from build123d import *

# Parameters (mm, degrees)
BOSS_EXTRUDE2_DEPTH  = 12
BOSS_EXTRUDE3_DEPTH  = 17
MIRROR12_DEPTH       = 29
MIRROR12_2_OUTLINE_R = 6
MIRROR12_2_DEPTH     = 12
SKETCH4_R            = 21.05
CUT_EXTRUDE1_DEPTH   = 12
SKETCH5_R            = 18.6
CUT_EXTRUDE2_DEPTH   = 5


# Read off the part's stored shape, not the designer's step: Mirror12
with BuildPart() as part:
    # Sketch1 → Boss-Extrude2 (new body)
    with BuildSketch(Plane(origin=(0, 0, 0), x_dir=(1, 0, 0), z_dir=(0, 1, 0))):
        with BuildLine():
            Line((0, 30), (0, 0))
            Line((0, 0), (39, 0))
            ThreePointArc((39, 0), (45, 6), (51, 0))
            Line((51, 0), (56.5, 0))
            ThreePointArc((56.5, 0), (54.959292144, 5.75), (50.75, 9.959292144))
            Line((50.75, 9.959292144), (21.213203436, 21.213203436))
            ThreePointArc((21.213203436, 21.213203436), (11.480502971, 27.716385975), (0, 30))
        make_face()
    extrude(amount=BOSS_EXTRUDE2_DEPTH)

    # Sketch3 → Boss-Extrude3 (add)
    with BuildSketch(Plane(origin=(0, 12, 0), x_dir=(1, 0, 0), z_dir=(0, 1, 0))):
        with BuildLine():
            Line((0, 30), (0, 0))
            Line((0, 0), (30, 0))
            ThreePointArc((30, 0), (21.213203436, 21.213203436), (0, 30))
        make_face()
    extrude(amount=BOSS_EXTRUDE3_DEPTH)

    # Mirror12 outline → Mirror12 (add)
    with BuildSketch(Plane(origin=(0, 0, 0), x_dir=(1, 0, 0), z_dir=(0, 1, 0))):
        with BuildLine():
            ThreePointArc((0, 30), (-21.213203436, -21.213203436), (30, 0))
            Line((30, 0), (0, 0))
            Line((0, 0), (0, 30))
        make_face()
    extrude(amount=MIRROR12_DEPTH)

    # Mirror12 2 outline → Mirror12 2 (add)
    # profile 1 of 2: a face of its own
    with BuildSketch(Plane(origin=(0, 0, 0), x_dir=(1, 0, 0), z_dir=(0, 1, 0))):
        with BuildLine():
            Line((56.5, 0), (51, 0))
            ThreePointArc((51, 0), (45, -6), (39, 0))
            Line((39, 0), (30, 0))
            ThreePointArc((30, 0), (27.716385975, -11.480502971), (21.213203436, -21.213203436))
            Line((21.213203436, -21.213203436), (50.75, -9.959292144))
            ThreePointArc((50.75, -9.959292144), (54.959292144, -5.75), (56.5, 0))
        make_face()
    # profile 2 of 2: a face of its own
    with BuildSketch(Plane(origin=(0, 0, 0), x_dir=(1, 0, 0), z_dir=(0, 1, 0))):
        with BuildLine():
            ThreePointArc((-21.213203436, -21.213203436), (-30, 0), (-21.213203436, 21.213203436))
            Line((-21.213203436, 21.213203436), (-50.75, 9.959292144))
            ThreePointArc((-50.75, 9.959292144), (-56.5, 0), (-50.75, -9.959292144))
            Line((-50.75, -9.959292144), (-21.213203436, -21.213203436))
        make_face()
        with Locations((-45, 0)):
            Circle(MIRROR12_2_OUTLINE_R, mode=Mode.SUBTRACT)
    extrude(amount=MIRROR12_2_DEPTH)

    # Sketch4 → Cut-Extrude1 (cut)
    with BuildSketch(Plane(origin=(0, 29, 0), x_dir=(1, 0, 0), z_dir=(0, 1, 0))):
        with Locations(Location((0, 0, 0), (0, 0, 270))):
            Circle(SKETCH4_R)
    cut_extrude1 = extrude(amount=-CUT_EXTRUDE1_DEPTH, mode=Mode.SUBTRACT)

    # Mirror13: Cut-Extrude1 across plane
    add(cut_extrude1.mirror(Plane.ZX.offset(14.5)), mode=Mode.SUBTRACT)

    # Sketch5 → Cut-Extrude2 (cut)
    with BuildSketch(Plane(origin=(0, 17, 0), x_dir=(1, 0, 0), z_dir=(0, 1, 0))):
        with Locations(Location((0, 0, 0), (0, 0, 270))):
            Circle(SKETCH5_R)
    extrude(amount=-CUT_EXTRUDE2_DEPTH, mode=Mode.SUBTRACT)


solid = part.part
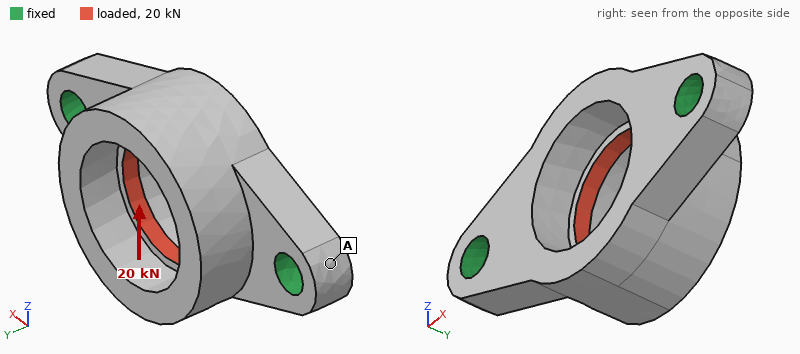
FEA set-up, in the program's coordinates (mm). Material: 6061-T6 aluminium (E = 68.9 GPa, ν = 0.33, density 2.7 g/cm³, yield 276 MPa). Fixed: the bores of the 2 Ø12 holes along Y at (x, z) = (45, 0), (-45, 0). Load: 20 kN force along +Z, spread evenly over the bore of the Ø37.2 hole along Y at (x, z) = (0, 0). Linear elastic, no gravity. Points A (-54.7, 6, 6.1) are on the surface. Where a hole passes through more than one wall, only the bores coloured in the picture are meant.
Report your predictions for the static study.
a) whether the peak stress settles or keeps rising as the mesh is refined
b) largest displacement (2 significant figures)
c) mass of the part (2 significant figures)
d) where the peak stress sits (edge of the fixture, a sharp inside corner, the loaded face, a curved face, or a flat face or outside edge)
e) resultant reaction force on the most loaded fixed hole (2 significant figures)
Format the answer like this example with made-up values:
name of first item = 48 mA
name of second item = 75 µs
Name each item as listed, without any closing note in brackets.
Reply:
whether the peak stress settles or keeps rising as the mesh is refined = keeps rising
largest displacement = 0.16 mm
mass of the part = 160 g
where the peak stress sits = edge of the fixture
resultant reaction force on the most loaded fixed hole = 10 kN
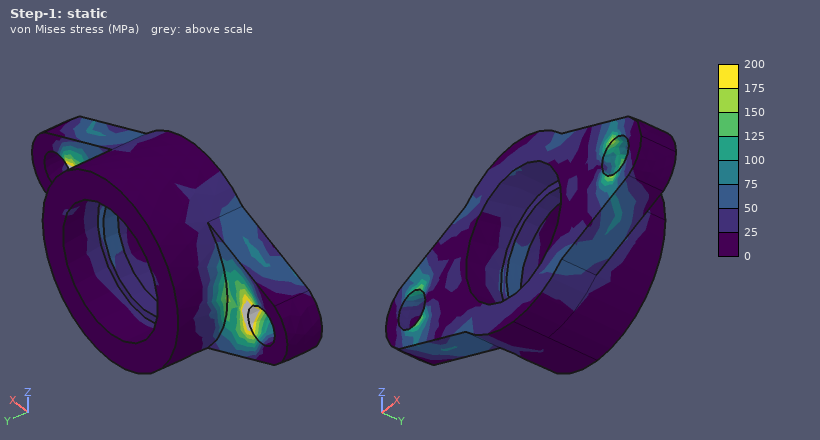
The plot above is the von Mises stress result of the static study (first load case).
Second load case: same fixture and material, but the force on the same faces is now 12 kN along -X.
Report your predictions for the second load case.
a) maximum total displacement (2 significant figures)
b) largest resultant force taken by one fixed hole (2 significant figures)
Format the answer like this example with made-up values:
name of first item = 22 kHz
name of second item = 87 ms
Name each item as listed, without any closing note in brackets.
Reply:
maximum total displacement = 15 µm
largest resultant force taken by one fixed hole = 6.1 kN
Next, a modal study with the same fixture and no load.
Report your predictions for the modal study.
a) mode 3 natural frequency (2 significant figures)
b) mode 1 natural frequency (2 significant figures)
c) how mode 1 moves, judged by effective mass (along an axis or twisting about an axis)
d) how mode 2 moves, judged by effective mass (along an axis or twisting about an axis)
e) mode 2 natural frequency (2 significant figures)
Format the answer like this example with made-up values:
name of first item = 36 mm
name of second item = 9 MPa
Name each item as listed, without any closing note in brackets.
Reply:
mode 3 natural frequency = 11 kHz
mode 1 natural frequency = 4600 Hz
how mode 1 moves, judged by effective mass = along Z
how mode 2 moves, judged by effective mass = along Y
mode 2 natural frequency = 6700 Hz
